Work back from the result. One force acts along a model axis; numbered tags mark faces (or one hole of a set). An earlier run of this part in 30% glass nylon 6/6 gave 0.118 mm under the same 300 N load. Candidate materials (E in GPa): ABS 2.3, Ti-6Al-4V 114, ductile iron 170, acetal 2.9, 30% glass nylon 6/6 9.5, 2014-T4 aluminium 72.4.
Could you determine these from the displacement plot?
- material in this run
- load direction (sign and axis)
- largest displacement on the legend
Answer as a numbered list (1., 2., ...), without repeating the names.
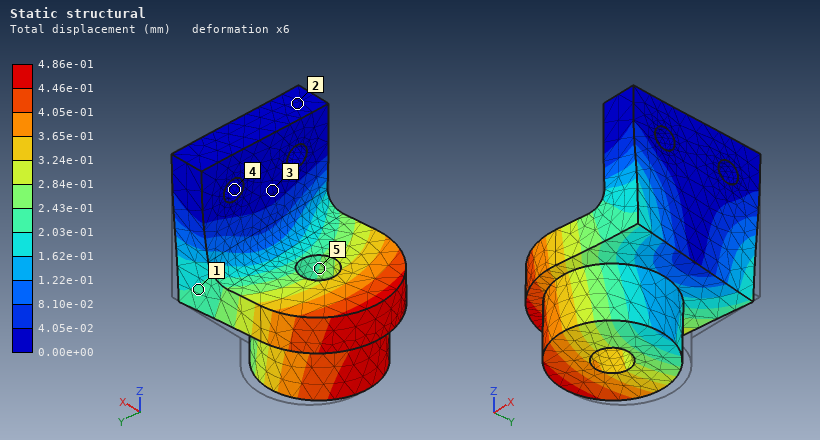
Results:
1. ABS
2. -Y
3. 4.86e-01 mm
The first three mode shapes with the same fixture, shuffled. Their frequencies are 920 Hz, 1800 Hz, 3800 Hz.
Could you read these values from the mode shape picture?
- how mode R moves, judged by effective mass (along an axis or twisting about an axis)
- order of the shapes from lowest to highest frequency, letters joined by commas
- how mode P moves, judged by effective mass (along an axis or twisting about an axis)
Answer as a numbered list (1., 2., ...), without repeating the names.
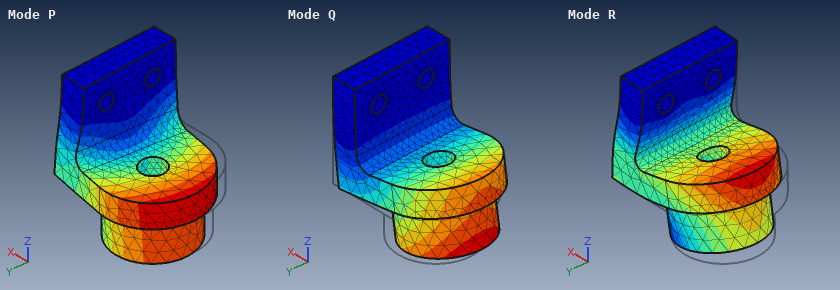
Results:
1. along X
2. Q, P, R
3. along Y
